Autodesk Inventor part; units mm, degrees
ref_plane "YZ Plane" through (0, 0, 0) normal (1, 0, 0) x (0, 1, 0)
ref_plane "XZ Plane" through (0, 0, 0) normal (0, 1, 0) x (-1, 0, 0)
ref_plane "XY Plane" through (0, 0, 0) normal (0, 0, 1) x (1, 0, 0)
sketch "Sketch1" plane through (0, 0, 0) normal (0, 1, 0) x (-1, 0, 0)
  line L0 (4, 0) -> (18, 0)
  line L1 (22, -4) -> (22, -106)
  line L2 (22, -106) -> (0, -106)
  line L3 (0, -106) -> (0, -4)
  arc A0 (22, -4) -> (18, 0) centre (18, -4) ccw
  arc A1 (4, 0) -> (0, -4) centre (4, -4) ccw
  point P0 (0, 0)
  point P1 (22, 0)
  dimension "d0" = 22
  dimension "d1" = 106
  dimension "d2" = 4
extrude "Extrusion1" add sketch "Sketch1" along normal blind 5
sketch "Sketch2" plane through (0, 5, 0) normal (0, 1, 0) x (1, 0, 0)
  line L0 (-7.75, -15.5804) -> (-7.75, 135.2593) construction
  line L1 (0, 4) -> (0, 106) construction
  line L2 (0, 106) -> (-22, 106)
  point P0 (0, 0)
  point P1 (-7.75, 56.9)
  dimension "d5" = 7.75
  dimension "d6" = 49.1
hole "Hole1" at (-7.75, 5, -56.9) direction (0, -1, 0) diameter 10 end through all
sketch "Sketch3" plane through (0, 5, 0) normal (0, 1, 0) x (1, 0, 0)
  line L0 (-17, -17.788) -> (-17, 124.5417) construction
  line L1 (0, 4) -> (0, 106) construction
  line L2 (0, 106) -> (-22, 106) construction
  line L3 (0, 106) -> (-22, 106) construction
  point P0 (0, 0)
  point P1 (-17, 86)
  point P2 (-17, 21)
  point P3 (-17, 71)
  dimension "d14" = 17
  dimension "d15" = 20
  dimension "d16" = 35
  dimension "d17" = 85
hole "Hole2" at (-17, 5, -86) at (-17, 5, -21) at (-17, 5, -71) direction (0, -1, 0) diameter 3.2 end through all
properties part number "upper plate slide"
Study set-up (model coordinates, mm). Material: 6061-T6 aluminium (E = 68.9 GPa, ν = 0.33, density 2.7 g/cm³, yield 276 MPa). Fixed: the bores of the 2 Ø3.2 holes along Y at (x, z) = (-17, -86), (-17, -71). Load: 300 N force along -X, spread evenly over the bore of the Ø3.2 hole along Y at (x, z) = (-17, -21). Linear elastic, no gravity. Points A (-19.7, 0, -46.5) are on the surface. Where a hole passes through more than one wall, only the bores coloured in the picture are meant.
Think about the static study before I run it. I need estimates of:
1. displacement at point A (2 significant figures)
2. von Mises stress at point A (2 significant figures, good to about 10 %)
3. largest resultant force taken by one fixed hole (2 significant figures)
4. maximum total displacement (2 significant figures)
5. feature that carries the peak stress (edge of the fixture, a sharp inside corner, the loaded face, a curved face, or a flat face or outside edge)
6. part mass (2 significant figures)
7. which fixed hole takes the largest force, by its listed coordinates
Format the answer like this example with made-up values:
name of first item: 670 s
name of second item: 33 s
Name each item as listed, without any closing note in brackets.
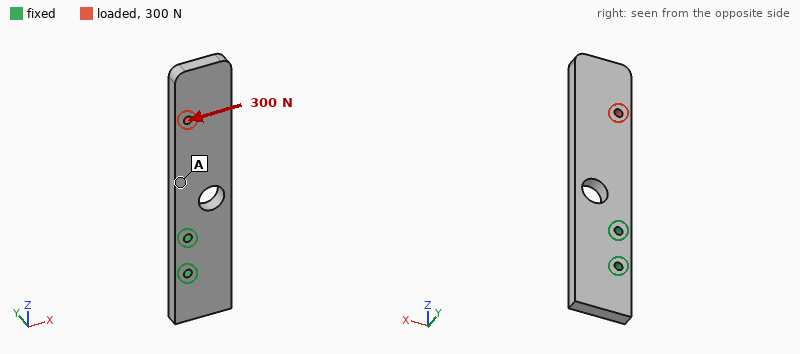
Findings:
displacement at point A: 0.037 mm
von Mises stress at point A: 12 MPa
largest resultant force taken by one fixed hole: 1.2 kN
maximum total displacement: 0.13 mm
feature that carries the peak stress: edge of the fixture
part mass: 30 g
which fixed hole takes the largest force, by its listed coordinates: (-17, -71)
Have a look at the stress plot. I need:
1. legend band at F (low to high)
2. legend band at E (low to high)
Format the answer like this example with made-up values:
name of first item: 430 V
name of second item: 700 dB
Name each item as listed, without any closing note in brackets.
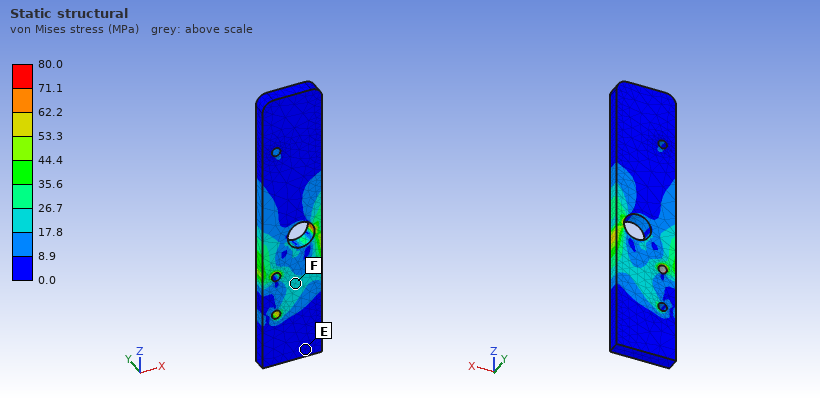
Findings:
legend band at F: 17.8 to 26.7 MPa
legend band at E: 0.0 to 8.9 MPa
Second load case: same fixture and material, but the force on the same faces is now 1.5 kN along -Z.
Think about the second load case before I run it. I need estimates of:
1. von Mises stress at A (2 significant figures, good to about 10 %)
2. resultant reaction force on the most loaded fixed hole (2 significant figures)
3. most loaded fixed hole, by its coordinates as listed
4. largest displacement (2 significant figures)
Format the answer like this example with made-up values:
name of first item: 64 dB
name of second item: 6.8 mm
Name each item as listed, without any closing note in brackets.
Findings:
von Mises stress at A: 33 MPa
resultant reaction force on the most loaded fixed hole: 1.3 kN
most loaded fixed hole, by its coordinates as listed: (-17, -71)
largest displacement: 65 µm
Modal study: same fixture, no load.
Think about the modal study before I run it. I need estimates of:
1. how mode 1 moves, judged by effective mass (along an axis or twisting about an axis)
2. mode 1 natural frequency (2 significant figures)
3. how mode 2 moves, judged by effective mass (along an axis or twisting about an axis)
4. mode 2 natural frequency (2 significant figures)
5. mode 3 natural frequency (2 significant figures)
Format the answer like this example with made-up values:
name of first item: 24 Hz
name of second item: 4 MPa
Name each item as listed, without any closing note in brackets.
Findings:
how mode 1 moves, judged by effective mass: along Y
mode 1 natural frequency: 700 Hz
how mode 2 moves, judged by effective mass: along X
mode 2 natural frequency: 2500 Hz
mode 3 natural frequency: 4000 Hz
